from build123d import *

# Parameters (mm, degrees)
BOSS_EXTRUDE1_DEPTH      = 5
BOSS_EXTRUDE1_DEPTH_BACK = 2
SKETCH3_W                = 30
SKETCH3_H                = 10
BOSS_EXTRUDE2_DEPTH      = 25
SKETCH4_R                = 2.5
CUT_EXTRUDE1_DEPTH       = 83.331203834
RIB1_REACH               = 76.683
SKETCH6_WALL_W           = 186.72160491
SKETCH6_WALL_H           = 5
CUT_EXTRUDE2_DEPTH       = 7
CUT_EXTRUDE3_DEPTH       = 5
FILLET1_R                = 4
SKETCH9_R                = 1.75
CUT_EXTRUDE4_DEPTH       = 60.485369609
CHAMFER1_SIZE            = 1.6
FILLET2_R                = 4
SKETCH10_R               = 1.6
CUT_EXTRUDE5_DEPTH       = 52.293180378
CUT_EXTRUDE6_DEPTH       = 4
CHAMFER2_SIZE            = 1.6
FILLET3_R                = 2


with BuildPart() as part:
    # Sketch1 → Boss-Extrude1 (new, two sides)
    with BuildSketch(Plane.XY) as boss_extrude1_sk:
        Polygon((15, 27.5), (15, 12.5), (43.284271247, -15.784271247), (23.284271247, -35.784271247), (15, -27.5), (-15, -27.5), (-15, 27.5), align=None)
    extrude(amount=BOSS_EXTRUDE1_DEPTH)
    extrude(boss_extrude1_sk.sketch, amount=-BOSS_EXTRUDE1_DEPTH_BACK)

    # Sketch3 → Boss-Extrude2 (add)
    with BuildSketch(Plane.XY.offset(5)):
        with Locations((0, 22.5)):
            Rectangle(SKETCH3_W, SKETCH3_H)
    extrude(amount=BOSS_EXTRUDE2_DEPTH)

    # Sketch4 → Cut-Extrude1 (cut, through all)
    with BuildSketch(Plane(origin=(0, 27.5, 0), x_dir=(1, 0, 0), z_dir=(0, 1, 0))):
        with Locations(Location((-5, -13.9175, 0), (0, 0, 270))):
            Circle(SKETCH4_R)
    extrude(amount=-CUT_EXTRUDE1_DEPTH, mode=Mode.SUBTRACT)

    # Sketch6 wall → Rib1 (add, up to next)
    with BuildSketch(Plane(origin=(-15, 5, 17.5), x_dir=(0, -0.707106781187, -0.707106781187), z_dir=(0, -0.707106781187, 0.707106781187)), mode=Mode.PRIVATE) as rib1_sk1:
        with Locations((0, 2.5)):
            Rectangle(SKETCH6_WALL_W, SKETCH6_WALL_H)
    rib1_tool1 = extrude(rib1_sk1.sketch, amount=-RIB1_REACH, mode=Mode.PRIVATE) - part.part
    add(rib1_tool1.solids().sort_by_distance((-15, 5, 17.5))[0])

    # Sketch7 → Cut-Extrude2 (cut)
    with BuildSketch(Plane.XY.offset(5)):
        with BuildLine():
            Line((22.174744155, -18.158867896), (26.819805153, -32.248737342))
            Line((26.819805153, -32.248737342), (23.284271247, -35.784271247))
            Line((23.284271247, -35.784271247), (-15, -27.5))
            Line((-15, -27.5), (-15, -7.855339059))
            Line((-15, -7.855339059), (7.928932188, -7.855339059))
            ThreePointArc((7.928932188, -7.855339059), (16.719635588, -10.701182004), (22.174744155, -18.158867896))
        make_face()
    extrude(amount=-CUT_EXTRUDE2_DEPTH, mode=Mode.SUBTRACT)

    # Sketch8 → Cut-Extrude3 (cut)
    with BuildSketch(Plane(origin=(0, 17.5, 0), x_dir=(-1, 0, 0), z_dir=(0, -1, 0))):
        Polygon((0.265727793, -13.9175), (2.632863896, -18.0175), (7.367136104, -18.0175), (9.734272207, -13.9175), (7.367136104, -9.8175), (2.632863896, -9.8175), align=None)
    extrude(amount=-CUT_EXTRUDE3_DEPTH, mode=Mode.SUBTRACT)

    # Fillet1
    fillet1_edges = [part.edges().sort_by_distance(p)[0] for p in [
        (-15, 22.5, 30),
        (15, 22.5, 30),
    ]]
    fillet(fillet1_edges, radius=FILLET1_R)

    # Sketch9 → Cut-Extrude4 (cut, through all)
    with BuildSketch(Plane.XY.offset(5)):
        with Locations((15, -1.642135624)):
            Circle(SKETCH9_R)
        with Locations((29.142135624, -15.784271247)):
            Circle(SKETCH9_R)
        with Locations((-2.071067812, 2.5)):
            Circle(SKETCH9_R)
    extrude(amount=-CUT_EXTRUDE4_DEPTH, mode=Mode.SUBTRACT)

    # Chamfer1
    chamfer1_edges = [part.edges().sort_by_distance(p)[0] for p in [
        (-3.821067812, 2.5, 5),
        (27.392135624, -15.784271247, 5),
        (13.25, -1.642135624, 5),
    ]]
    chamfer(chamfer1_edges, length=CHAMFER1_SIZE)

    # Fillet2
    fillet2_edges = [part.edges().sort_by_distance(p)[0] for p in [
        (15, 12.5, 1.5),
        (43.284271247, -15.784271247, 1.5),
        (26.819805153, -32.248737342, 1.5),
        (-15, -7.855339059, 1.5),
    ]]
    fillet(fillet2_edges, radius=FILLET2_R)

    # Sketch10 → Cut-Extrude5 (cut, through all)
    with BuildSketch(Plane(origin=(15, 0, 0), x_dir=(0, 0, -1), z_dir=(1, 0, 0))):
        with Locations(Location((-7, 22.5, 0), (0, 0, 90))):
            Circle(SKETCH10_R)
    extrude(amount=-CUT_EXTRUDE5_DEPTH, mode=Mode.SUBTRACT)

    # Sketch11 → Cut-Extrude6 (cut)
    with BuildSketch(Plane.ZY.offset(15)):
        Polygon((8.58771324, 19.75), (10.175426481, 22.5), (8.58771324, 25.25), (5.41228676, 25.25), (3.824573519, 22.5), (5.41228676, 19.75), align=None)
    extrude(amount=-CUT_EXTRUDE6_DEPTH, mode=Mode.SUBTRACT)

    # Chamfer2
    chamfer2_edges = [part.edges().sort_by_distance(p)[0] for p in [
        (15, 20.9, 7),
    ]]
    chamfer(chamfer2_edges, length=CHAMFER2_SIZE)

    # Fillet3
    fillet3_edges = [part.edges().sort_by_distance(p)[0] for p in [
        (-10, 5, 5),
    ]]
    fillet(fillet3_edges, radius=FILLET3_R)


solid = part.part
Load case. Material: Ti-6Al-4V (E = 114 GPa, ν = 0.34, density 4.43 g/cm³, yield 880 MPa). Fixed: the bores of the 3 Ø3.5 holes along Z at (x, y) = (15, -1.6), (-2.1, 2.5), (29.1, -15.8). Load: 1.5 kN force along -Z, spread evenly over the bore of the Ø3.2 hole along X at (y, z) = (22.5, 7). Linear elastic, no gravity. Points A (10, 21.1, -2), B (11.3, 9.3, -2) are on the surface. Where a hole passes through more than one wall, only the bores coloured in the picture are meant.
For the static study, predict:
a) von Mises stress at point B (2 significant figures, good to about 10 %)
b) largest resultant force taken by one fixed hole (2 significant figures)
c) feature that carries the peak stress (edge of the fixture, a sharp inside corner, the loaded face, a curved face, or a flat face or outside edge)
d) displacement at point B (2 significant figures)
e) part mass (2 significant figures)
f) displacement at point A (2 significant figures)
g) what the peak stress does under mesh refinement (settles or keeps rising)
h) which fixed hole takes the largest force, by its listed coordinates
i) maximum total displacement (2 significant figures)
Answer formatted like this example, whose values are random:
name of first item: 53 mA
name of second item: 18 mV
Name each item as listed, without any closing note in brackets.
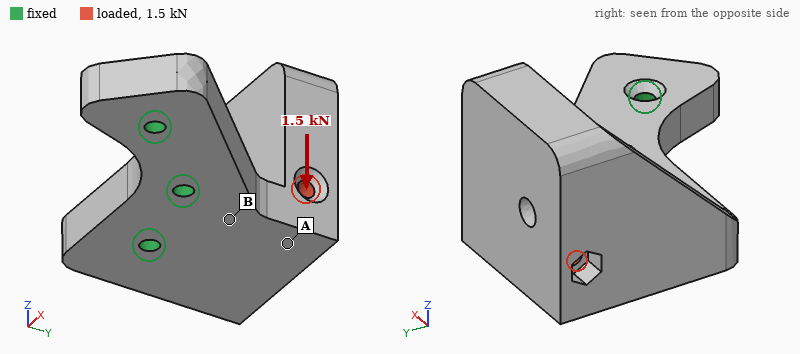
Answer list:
von Mises stress at point B: 54 MPa
largest resultant force taken by one fixed hole: 1.3 kN
feature that carries the peak stress: edge of the fixture
displacement at point B: 0.017 mm
part mass: 85 g
displacement at point A: 0.050 mm
what the peak stress does under mesh refinement: keeps rising
which fixed hole takes the largest force, by its listed coordinates: (-2.1, 2.5)
maximum total displacement: 0.11 mm
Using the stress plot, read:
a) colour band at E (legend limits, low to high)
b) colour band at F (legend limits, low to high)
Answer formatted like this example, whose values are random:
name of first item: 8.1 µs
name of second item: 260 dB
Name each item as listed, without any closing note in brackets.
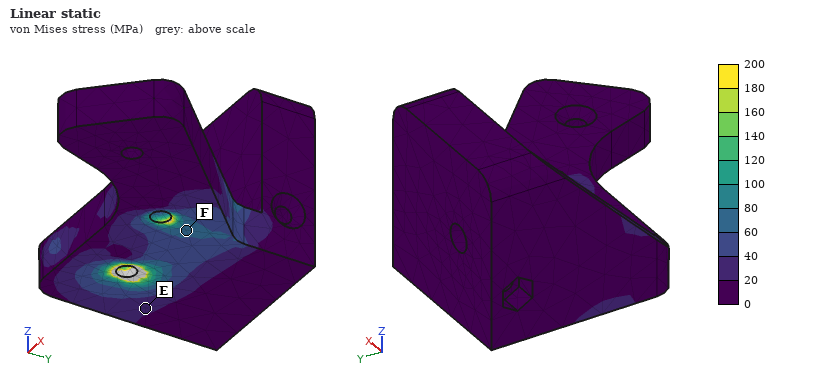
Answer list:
colour band at E: 20 to 40 MPa
colour band at F: 60 to 80 MPa
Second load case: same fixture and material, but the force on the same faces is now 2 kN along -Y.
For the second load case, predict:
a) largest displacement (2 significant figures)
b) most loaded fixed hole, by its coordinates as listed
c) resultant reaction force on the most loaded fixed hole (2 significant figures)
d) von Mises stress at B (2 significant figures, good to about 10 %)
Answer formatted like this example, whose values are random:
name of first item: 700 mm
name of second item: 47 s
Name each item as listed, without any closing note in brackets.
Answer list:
largest displacement: 53 µm
most loaded fixed hole, by its coordinates as listed: (-2.1, 2.5)
resultant reaction force on the most loaded fixed hole: 1.5 kN
von Mises stress at B: 19 MPa
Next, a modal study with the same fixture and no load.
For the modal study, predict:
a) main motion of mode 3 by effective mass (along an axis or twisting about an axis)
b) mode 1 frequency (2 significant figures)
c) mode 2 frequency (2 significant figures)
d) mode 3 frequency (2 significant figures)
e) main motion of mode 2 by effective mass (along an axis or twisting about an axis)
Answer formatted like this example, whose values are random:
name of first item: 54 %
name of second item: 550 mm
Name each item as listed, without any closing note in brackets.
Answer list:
main motion of mode 3 by effective mass: along Z
mode 1 frequency: 2900 Hz
mode 2 frequency: 4400 Hz
mode 3 frequency: 10 kHz
main motion of mode 2 by effective mass: along X
